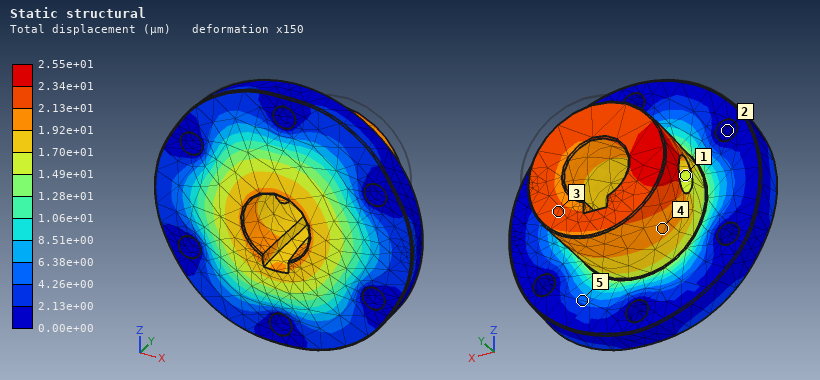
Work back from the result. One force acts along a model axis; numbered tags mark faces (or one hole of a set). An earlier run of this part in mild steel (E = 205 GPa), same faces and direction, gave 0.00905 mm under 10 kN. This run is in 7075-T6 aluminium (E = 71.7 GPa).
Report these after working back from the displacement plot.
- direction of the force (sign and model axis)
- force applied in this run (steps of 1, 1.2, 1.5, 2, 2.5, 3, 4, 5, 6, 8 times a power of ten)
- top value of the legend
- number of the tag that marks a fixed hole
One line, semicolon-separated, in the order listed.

-Y; 10 kN; 2.55e+01 µm; 2
